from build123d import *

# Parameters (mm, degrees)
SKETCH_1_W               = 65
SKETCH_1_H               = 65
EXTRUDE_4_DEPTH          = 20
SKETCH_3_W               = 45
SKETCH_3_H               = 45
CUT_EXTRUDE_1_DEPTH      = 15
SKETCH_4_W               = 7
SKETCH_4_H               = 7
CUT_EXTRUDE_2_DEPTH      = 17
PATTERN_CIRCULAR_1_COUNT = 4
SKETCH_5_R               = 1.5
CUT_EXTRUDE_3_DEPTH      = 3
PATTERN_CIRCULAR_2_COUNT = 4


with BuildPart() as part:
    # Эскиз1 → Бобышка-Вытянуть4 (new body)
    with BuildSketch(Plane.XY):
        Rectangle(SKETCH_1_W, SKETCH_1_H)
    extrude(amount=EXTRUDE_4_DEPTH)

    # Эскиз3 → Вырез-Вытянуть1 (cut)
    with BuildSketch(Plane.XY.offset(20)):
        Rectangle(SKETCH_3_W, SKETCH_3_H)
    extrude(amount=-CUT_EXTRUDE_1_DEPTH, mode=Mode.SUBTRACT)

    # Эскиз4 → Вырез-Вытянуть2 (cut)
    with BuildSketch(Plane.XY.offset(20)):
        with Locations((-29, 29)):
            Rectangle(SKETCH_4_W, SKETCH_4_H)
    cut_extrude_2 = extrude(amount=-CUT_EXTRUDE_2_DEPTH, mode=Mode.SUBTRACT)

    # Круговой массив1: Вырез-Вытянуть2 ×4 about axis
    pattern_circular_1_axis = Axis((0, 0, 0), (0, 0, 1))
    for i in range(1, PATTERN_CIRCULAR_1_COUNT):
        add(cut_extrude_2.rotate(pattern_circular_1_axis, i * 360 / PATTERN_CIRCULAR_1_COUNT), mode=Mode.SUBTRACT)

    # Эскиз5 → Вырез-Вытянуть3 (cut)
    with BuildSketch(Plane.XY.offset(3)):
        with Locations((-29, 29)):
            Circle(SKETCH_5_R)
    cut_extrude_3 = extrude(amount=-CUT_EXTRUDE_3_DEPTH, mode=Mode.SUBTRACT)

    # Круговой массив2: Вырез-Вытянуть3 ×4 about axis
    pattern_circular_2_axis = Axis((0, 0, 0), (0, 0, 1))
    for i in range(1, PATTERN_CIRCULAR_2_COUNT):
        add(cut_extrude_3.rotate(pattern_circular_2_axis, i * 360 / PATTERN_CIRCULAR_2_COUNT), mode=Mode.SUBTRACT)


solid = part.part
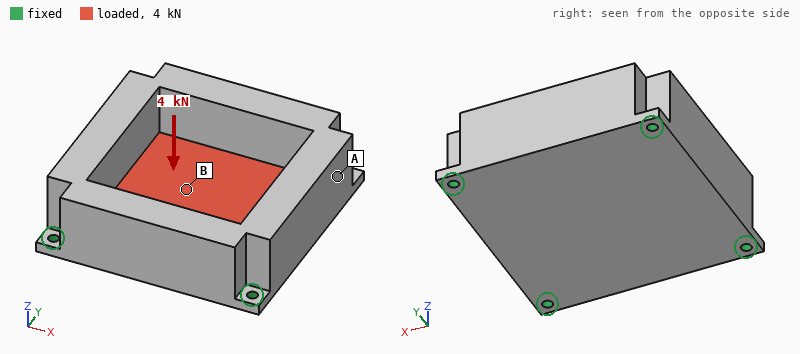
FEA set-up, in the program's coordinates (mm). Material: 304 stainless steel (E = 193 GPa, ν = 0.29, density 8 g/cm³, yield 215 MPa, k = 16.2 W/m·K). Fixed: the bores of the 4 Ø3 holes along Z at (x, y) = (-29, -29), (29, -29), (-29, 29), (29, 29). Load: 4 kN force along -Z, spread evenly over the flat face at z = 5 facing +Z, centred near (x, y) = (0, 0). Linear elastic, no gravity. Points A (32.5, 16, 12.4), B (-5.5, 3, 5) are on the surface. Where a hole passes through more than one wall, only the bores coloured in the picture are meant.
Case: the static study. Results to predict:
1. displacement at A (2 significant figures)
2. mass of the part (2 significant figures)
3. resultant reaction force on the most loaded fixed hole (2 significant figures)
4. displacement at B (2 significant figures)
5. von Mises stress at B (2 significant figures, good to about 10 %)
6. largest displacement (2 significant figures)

3.9 µm
410 g
1.2 kN
15 µm
24 MPa
16 µm
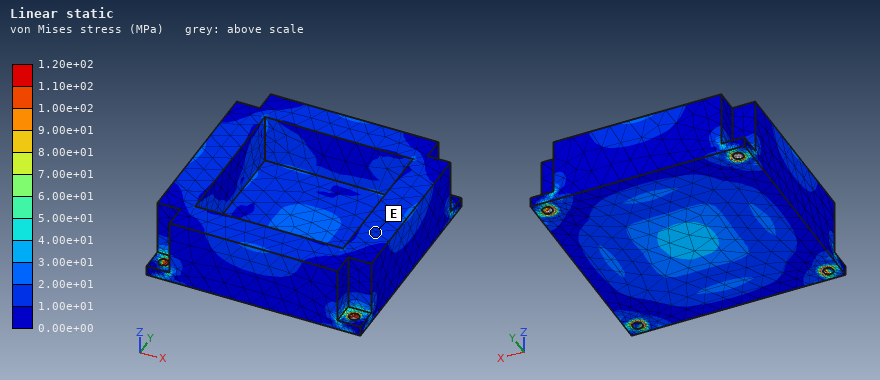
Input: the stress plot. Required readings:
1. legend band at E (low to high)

1.00e+01 to 2.00e+01 MPa
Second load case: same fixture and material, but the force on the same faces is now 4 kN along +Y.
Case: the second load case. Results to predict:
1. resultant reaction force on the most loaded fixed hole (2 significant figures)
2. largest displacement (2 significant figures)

1.1 kN
3.0 µm
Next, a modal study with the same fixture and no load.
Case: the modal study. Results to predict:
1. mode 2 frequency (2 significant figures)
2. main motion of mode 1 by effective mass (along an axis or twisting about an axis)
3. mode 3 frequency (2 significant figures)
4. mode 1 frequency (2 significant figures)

9600 Hz
along Z
9600 Hz
7400 Hz
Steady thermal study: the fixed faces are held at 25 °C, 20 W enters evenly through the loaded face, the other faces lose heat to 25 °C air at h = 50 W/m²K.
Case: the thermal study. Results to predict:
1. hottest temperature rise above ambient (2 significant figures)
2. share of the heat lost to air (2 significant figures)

39 K
66 %
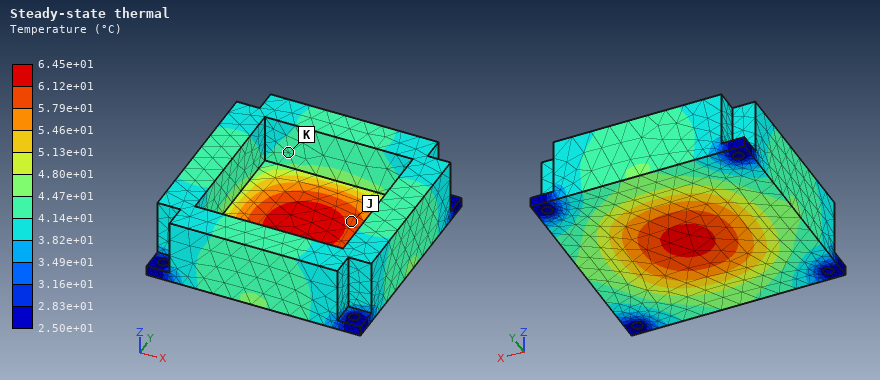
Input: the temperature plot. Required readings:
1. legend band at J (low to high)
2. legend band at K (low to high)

5.79e+01 to 6.12e+01 °C
4.14e+01 to 4.47e+01 °C
